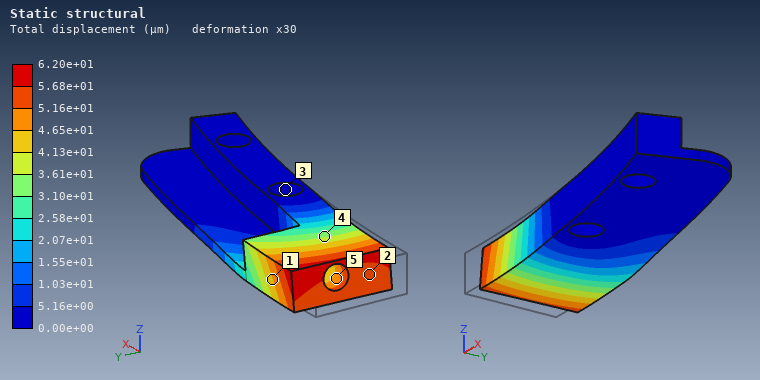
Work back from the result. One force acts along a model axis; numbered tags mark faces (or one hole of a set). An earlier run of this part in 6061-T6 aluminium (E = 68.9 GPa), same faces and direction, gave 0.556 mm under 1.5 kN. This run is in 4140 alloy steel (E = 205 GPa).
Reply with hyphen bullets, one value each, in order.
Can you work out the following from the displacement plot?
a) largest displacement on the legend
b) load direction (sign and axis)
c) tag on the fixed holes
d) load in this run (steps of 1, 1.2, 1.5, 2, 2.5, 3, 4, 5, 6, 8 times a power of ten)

- 6.20e+01 µm
- +Y
- 3
- 500 N
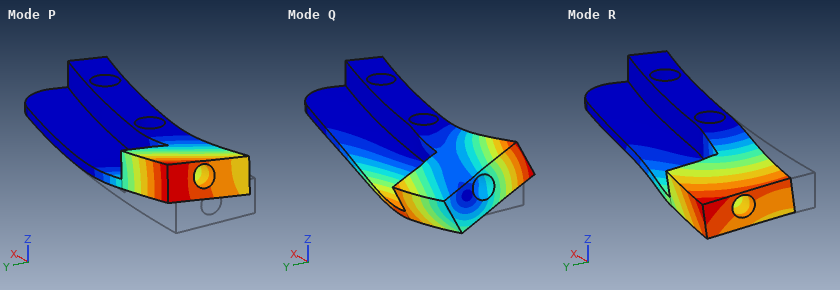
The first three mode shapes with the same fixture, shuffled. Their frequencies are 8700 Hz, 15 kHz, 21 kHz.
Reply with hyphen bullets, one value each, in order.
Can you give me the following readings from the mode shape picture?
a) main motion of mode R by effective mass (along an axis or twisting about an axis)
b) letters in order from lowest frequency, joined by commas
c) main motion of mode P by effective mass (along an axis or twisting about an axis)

- along Y
- P, R, Q
- along Z
